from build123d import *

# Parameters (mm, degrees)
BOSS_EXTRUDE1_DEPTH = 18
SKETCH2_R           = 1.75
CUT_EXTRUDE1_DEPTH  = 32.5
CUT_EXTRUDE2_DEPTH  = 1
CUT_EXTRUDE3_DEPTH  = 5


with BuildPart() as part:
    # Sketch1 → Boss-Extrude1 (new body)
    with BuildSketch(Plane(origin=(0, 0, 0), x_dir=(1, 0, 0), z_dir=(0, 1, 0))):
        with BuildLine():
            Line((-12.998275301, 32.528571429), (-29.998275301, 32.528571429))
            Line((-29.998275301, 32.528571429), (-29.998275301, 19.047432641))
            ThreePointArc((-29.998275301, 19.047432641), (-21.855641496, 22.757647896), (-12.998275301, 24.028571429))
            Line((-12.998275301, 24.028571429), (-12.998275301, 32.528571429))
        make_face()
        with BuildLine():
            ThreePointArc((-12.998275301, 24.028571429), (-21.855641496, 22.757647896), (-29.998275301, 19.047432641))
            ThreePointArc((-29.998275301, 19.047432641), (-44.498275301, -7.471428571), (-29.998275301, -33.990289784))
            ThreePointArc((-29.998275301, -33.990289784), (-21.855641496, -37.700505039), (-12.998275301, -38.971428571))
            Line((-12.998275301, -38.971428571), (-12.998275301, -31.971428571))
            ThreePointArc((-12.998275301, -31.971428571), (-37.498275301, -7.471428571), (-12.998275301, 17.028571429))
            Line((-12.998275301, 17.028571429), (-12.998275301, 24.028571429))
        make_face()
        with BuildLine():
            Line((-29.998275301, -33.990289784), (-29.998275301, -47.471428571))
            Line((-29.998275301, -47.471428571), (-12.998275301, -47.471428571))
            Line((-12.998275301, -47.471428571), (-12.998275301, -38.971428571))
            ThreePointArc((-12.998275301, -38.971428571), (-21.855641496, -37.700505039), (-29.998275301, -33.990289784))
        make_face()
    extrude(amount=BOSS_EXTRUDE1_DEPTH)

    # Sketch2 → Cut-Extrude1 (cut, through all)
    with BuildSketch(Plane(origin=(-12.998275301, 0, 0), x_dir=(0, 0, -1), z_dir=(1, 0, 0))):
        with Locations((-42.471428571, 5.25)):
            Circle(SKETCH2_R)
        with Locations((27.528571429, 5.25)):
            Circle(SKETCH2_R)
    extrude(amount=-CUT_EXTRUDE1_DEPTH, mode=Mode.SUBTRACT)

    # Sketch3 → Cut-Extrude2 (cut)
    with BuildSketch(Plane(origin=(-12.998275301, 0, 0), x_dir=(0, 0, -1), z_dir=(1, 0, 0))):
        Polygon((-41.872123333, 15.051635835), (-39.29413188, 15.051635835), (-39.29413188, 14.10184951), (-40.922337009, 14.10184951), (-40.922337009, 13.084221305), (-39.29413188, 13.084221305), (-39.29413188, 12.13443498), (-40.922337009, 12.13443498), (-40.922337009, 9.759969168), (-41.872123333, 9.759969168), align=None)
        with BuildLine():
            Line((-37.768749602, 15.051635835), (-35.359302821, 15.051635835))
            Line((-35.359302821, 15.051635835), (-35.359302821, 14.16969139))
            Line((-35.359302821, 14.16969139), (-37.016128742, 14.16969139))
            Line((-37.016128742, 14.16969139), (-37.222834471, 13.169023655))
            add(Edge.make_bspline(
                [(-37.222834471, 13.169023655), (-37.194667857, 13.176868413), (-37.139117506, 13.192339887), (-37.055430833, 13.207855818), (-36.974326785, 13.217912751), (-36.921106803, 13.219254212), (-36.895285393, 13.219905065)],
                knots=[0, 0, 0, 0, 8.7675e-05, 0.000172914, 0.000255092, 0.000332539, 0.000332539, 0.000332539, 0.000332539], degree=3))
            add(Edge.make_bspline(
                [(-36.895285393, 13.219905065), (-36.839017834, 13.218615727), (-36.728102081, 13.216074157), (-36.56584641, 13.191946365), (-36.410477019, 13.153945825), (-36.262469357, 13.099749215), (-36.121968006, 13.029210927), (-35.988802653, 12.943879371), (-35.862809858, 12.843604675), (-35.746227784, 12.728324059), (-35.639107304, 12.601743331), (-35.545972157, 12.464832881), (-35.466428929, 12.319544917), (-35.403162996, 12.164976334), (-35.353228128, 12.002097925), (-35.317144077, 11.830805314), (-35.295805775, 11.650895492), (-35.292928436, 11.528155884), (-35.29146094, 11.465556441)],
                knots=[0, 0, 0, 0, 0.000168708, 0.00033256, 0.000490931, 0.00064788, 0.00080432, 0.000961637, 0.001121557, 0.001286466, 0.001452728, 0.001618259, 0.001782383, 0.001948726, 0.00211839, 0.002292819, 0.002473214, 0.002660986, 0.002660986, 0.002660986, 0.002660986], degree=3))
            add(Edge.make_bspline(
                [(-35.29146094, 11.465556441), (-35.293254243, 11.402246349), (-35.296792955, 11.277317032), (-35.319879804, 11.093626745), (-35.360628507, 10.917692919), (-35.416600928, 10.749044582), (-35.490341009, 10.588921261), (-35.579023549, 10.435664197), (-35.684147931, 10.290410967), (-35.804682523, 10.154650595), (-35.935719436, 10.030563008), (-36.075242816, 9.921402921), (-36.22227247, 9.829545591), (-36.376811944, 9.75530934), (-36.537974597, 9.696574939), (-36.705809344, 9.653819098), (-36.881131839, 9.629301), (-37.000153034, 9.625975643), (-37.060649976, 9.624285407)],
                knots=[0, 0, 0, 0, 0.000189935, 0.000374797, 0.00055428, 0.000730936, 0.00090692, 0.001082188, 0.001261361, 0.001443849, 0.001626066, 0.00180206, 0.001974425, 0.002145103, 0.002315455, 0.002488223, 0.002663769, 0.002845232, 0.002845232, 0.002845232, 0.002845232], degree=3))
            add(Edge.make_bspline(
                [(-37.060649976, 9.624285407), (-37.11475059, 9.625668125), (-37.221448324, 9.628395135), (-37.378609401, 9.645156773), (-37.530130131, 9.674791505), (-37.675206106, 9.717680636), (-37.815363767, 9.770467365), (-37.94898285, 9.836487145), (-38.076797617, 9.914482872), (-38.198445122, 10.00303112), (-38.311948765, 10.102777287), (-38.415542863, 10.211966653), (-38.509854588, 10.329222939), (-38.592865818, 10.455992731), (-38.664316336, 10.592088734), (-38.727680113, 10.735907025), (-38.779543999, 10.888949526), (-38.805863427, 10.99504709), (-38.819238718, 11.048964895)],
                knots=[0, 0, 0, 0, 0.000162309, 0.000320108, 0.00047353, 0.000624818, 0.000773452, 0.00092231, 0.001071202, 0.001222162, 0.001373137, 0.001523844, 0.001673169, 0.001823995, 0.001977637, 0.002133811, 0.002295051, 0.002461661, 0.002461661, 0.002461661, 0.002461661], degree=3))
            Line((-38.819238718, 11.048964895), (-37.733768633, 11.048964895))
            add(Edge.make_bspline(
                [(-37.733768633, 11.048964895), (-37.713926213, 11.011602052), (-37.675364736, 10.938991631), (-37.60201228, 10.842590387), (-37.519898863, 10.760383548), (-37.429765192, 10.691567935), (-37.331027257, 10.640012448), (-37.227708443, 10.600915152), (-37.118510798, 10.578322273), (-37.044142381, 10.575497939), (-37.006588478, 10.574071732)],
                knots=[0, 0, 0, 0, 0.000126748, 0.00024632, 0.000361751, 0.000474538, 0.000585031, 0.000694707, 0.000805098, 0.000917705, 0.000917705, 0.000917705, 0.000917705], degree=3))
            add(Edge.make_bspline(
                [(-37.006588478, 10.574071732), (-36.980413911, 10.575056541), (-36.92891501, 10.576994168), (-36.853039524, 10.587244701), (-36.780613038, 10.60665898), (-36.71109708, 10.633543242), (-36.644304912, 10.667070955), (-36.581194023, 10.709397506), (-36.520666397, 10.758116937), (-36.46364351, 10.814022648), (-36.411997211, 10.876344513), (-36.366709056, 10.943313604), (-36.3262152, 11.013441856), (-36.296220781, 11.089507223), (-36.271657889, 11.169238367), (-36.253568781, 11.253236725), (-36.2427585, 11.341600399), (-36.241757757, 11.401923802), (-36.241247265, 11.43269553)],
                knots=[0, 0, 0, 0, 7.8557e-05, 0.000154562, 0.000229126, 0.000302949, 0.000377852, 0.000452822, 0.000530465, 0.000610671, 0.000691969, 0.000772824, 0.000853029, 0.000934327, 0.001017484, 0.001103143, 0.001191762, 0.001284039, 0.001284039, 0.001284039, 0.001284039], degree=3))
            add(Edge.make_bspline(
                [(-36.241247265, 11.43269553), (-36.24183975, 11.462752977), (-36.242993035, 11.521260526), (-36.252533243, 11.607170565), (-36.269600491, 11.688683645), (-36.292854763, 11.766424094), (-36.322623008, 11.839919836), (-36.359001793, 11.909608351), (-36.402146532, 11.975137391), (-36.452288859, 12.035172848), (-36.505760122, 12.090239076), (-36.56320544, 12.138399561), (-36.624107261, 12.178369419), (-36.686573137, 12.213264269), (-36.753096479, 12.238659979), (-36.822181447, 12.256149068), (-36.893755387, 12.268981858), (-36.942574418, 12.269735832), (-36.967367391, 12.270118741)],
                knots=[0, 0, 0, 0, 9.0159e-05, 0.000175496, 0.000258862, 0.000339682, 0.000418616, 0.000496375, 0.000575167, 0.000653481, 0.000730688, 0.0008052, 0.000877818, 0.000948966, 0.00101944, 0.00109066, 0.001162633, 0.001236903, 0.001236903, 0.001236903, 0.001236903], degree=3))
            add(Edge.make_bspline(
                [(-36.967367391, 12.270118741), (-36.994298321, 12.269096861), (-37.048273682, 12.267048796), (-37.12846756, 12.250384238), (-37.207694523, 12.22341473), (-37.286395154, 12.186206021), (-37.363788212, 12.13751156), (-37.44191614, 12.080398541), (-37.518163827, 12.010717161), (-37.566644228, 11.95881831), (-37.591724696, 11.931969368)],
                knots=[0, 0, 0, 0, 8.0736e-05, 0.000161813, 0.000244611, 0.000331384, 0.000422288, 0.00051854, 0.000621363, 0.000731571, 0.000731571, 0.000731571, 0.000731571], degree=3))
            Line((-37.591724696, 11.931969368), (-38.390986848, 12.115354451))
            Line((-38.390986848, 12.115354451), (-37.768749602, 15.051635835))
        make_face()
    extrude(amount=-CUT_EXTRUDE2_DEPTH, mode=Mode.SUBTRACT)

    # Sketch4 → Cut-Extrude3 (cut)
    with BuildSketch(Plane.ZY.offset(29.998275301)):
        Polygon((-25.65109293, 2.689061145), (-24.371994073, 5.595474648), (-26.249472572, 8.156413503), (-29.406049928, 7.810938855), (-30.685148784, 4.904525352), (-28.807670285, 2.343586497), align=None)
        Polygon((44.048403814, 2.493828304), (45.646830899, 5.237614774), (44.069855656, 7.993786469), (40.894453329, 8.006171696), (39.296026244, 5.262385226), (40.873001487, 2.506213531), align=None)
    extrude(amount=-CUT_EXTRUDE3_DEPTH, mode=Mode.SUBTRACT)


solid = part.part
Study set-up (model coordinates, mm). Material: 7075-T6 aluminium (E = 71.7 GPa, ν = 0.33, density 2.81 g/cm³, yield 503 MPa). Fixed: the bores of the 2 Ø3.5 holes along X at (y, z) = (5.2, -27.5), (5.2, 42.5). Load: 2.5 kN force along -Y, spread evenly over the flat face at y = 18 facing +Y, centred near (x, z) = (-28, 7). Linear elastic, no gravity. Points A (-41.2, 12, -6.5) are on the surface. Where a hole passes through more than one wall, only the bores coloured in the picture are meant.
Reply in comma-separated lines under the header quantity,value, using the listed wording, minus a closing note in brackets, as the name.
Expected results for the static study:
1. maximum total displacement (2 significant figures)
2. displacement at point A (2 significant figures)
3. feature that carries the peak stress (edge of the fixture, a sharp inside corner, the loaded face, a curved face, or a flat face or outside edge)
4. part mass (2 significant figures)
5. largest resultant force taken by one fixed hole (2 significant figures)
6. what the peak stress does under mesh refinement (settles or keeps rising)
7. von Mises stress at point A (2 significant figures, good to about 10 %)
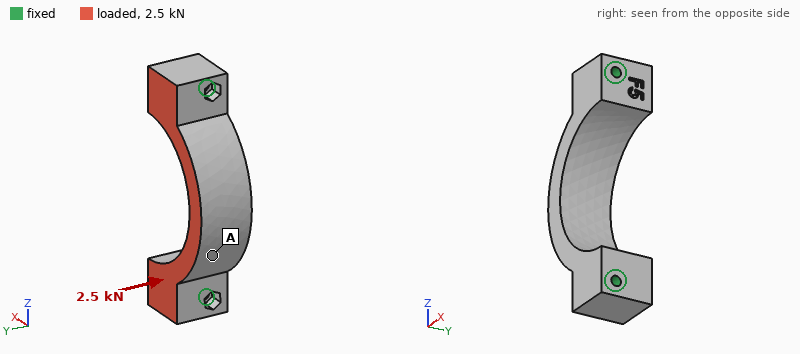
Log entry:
quantity,value
maximum total displacement,47 µm
displacement at point A,36 µm
feature that carries the peak stress,edge of the fixture
part mass,47 g
largest resultant force taken by one fixed hole,1.3 kN
what the peak stress does under mesh refinement,keeps rising
von Mises stress at point A,16 MPa
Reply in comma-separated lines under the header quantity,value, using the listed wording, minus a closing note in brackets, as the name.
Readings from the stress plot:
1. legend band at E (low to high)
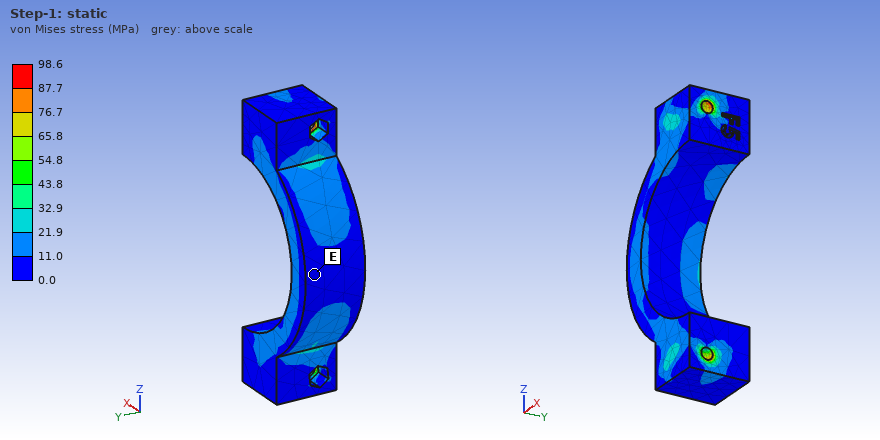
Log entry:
quantity,value
legend band at E,0.0 to 11.0 MPa
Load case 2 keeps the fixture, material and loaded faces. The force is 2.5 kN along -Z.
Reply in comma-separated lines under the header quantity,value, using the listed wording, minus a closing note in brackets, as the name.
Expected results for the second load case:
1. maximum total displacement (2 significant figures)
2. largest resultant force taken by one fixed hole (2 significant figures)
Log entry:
quantity,value
maximum total displacement,13 µm
largest resultant force taken by one fixed hole,1.3 kN
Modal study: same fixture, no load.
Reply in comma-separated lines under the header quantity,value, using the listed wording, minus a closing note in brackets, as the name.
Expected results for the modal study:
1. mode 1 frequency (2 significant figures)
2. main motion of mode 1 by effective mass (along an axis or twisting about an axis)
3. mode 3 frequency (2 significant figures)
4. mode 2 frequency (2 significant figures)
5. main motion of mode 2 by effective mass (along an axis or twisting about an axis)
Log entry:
quantity,value
mode 1 frequency,6500 Hz
main motion of mode 1 by effective mass,along Y
mode 3 frequency,17 kHz
mode 2 frequency,13 kHz
main motion of mode 2 by effective mass,along Z
